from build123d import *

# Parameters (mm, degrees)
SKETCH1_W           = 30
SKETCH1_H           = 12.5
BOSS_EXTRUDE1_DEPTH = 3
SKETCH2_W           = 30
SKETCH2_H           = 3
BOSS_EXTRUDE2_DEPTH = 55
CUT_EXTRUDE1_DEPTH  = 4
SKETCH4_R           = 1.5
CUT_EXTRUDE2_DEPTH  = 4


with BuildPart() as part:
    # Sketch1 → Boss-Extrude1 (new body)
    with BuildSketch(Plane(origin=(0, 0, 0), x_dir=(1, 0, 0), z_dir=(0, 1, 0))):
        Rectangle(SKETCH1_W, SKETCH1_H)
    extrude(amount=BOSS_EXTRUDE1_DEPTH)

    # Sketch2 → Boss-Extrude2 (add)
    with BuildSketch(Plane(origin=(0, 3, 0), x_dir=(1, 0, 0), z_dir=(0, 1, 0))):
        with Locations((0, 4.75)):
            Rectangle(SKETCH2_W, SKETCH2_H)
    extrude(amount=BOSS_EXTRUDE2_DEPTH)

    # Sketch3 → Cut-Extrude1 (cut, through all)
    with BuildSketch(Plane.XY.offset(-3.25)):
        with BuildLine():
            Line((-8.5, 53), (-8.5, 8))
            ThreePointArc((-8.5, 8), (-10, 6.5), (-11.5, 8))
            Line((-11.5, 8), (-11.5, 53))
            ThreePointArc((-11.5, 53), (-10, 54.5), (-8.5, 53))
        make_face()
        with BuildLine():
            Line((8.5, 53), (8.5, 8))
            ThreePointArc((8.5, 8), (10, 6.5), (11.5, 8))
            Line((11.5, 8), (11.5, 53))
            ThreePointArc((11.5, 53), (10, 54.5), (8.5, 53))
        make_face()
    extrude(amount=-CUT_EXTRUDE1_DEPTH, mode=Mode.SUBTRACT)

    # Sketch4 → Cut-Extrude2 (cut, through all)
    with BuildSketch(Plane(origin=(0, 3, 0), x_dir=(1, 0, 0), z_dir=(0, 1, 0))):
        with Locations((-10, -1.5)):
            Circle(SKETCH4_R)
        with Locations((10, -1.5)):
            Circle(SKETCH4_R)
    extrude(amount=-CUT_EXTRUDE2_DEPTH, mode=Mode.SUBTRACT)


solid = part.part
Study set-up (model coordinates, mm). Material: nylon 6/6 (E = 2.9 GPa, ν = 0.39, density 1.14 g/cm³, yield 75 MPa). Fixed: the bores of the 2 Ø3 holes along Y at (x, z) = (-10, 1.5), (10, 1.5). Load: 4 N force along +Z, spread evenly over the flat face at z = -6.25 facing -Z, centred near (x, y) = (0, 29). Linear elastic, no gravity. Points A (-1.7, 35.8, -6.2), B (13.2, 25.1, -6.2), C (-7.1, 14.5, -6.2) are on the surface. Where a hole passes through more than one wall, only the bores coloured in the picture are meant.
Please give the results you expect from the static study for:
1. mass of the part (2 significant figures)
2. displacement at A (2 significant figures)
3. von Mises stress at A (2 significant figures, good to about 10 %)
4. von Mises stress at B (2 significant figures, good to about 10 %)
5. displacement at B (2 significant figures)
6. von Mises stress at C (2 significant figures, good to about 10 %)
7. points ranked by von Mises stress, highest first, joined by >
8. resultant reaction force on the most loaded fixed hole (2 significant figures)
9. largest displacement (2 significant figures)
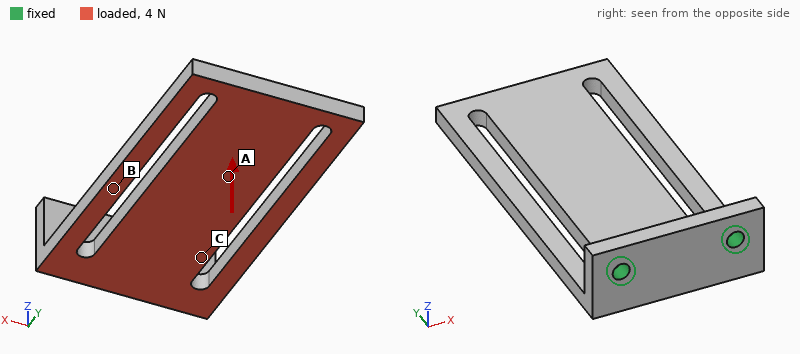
5.9 g
0.34 mm
0.49 MPa
1.1 MPa
0.19 mm
1.8 MPa
C > B > A
2.2 N
0.67 mm
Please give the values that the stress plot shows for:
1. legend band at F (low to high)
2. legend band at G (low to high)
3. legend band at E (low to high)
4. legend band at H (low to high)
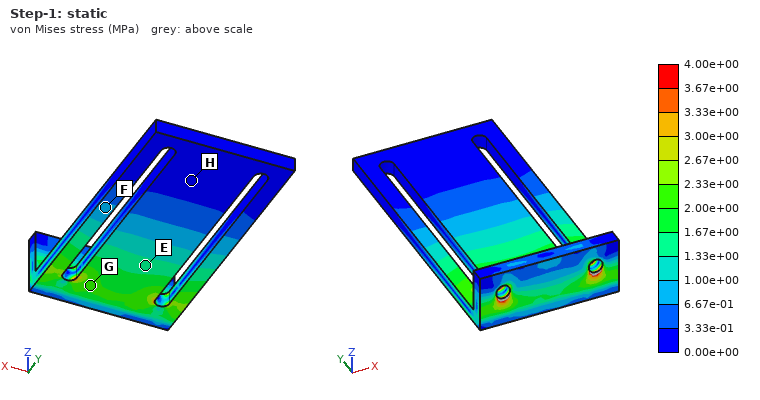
6.67e-01 to 1.00e+00 MPa
2.00e+00 to 2.33e+00 MPa
1.33e+00 to 1.67e+00 MPa
0.00e+00 to 3.33e-01 MPa
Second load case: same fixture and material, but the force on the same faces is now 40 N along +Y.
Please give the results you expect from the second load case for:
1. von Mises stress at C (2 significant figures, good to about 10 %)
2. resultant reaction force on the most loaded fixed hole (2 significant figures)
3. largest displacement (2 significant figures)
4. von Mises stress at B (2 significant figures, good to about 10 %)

1.7 MPa
20 N
0.69 mm
1.3 MPa
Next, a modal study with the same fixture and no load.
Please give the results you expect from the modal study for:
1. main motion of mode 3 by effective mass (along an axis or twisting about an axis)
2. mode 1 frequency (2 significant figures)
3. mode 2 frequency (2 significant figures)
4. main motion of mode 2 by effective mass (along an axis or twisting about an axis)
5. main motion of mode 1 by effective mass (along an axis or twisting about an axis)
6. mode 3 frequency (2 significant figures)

along X
210 Hz
780 Hz
along X
along Z
950 Hz
